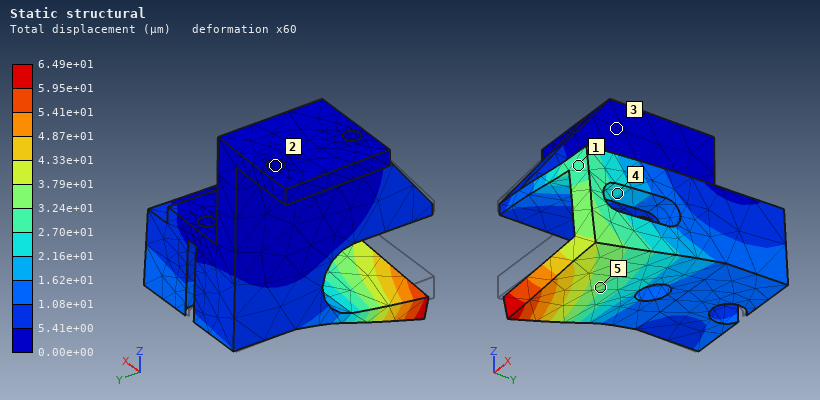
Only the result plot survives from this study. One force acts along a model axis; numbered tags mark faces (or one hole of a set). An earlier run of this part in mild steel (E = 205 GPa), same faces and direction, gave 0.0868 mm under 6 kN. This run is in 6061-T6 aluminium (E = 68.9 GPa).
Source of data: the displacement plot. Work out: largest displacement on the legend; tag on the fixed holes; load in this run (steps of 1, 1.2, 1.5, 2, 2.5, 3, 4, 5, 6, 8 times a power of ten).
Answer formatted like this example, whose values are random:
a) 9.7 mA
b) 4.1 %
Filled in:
a) 6.49e+01 µm
b) 2
c) 1.5 kN
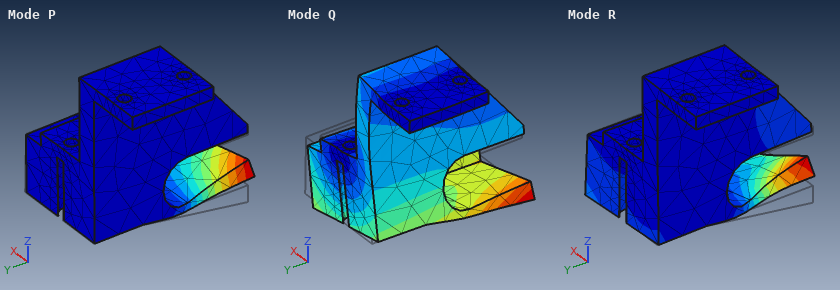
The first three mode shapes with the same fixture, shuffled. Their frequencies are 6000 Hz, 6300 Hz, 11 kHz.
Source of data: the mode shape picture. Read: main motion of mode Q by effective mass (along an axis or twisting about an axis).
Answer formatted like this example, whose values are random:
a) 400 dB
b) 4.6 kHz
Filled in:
a) along X
